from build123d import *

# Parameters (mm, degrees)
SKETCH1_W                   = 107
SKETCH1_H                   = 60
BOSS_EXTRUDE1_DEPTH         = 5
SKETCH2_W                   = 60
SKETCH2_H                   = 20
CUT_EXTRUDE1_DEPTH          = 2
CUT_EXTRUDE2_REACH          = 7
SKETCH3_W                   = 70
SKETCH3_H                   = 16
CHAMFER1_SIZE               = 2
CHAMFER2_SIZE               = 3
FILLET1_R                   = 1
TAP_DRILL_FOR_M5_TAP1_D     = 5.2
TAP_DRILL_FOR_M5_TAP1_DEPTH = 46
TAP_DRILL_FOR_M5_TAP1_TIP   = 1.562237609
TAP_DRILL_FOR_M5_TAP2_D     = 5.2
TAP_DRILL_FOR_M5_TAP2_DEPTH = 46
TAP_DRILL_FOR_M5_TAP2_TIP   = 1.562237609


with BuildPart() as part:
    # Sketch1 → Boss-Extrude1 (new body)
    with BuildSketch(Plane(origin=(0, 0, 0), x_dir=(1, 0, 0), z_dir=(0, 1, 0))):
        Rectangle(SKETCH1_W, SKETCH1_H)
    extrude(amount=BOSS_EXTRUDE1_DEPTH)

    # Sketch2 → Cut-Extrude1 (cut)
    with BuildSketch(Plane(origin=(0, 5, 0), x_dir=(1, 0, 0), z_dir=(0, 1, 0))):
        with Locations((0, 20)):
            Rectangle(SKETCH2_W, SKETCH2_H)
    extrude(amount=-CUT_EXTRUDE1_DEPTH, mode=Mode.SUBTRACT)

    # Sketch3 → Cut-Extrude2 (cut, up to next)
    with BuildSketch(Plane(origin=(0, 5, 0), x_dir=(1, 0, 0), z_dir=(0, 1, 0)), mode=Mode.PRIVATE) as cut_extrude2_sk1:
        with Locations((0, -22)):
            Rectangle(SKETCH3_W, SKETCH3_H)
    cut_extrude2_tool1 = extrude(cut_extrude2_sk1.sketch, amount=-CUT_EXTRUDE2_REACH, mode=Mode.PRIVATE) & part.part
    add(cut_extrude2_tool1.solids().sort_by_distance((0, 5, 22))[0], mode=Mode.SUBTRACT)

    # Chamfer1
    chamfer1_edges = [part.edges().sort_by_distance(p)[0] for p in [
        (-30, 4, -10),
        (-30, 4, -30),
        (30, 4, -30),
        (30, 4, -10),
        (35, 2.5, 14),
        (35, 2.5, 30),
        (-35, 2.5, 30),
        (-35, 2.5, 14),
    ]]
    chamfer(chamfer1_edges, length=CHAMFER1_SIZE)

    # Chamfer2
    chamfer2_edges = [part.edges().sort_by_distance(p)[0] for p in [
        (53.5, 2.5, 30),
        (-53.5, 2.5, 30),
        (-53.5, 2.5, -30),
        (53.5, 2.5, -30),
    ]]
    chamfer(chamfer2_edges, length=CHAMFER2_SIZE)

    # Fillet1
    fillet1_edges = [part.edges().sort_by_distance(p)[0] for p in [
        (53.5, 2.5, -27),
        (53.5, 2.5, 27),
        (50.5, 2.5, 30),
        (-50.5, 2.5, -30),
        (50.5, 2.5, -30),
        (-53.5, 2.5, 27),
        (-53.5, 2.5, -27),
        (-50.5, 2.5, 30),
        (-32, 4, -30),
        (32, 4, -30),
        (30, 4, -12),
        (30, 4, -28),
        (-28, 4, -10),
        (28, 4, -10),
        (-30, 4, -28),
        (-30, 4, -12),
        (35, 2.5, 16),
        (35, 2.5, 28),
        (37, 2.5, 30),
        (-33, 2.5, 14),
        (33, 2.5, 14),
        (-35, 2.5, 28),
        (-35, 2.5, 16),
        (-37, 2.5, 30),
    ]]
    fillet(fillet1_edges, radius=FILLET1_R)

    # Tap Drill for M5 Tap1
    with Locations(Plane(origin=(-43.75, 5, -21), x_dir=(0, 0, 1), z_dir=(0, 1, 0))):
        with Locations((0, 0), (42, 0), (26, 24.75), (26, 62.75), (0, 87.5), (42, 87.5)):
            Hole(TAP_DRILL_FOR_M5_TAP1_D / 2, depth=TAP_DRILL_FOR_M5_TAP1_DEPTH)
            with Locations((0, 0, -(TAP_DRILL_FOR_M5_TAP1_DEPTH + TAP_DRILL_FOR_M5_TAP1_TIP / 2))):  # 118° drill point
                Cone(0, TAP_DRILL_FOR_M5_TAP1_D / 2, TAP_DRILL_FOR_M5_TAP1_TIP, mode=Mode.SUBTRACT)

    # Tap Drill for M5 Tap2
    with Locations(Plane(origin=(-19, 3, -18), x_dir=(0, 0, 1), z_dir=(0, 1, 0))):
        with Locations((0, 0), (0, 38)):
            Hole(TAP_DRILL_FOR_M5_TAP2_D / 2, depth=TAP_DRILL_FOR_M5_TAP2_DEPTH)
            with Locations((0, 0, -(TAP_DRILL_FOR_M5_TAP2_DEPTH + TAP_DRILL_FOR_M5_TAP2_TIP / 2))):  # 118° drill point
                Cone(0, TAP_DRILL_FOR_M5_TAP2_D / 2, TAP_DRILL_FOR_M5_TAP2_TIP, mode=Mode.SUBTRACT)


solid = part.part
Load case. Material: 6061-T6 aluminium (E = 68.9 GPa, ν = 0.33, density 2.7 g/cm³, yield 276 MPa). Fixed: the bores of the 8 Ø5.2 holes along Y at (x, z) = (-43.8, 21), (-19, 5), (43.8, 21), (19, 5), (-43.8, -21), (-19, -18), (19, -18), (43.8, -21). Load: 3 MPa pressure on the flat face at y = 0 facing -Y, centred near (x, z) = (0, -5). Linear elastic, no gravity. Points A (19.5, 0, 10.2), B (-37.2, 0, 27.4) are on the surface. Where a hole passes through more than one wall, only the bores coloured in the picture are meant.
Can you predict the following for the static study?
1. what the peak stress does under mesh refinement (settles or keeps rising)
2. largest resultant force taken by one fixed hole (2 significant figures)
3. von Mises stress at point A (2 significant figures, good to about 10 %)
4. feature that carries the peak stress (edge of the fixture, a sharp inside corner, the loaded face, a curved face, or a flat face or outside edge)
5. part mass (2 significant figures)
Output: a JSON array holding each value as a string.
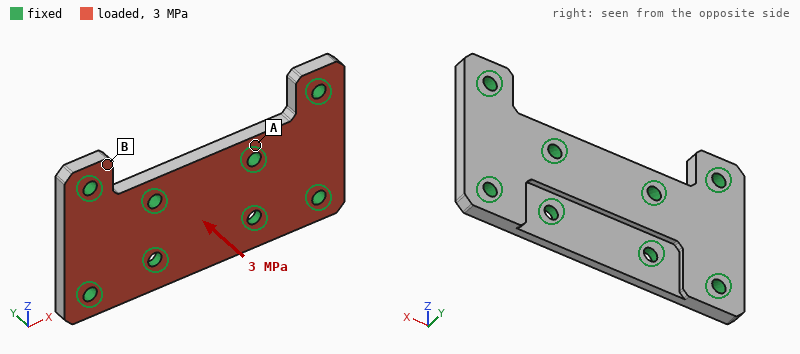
["keeps rising", "2.2 kN", "37 MPa", "edge of the fixture", "63 g"]
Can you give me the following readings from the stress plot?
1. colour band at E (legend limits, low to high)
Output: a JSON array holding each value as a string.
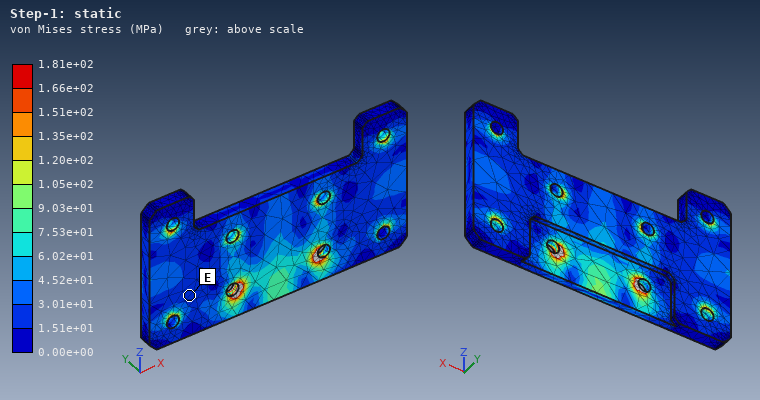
["1.51e+01 to 3.01e+01 MPa"]
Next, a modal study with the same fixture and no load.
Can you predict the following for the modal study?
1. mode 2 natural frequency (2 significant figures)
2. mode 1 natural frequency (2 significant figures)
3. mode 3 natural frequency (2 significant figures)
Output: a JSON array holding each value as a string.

["15 kHz", "11 kHz", "15 kHz"]
